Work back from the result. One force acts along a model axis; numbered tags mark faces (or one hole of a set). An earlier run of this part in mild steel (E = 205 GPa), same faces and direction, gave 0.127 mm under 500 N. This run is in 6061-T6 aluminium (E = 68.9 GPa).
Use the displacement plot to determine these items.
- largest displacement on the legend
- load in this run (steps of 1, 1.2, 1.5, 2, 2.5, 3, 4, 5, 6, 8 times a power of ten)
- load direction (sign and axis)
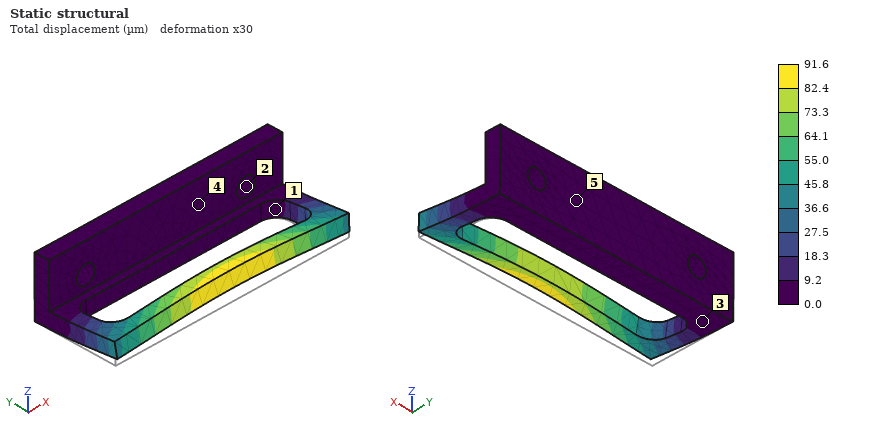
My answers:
91.6 µm
120 N
+Z
